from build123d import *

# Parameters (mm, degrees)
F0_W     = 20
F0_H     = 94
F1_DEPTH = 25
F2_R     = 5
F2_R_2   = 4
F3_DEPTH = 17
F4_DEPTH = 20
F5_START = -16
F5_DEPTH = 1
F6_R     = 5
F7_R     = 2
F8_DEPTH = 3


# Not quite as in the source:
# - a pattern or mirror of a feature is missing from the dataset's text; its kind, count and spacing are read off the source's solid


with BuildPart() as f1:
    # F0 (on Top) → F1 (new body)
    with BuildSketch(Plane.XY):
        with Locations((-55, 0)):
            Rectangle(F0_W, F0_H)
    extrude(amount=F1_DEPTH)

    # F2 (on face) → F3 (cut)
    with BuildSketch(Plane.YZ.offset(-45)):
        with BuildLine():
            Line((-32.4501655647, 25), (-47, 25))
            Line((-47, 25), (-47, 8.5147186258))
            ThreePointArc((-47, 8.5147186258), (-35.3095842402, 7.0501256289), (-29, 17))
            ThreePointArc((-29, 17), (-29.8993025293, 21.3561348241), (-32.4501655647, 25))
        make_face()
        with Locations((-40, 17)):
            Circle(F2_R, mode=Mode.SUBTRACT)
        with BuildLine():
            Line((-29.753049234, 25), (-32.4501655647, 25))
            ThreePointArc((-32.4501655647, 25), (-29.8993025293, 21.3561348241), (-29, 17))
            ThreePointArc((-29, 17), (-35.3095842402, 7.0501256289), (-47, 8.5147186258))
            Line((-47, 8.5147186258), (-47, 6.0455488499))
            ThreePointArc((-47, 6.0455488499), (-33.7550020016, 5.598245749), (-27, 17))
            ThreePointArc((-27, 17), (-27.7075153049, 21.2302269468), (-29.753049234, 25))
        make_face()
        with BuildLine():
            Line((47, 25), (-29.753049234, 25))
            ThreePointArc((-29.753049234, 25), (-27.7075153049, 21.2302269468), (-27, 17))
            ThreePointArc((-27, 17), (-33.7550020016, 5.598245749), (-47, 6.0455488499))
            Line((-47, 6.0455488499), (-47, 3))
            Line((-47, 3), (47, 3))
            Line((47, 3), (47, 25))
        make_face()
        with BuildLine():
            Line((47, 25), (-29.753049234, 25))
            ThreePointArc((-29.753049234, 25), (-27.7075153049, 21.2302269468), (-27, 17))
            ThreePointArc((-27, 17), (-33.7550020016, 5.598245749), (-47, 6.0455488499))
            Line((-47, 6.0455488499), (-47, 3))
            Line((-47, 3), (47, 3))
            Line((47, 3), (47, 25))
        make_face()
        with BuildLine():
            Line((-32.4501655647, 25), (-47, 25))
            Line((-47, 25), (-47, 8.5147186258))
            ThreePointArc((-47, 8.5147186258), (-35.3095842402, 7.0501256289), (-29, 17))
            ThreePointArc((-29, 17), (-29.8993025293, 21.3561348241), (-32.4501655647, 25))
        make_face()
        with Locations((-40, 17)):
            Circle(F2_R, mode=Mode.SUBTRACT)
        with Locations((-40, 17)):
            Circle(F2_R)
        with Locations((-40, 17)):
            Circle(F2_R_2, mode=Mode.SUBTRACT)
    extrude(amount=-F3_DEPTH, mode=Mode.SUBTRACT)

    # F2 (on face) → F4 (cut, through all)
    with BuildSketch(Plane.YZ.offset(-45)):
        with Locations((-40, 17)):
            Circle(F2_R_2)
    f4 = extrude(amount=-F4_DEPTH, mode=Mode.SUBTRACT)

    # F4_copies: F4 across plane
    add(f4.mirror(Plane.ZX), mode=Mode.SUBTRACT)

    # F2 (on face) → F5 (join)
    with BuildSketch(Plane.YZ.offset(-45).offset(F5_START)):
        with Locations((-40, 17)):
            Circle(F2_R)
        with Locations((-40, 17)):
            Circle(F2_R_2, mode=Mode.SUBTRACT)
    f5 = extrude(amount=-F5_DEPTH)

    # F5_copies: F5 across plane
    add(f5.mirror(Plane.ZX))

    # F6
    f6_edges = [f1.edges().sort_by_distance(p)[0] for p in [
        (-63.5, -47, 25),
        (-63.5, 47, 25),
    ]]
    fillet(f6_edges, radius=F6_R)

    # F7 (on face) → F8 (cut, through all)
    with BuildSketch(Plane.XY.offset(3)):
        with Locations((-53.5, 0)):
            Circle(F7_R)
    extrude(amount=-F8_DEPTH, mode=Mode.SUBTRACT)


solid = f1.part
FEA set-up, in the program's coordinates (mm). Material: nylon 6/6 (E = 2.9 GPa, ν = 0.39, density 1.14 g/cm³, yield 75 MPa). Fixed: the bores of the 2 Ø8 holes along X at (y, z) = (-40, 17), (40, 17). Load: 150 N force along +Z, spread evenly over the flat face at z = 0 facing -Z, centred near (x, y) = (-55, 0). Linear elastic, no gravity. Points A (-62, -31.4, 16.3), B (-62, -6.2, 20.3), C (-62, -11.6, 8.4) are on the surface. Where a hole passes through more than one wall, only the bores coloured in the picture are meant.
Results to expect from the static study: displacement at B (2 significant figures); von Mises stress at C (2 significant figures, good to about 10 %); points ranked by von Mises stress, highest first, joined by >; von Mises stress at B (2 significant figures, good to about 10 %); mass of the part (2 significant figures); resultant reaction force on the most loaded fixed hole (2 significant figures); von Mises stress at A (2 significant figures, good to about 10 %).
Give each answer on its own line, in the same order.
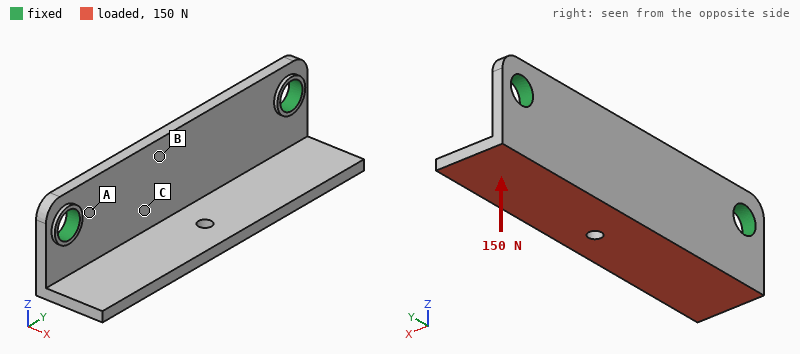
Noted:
0.30 mm
5.6 MPa
A > C > B
2.9 MPa
13 g
79 N
9.1 MPa
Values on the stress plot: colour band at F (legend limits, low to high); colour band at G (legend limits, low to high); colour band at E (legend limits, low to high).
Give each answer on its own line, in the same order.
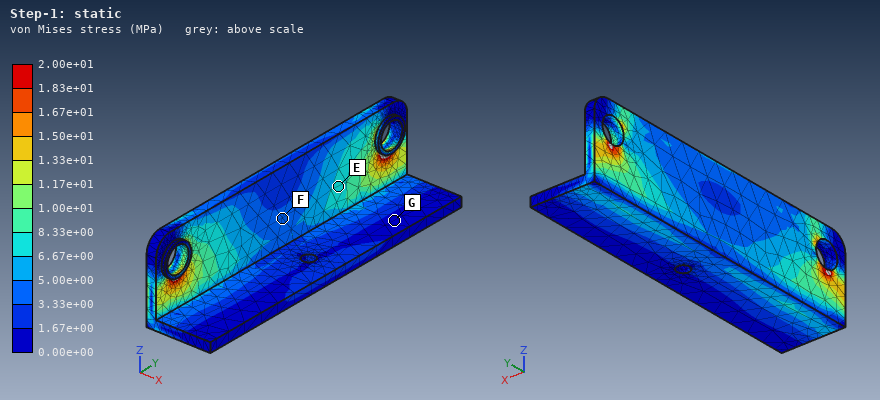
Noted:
3.33e+00 to 5.00e+00 MPa
0.00e+00 to 1.67e+00 MPa
6.67e+00 to 8.33e+00 MPa
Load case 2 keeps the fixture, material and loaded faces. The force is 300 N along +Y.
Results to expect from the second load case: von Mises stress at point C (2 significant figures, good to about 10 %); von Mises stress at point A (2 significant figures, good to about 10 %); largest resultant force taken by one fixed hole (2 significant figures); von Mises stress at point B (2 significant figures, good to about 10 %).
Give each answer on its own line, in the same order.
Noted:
2.6 MPa
3.6 MPa
160 N
1.3 MPa
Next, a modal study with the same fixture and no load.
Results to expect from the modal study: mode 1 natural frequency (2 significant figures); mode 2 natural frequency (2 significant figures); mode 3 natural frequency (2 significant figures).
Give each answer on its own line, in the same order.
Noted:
830 Hz
1300 Hz
1300 Hz
